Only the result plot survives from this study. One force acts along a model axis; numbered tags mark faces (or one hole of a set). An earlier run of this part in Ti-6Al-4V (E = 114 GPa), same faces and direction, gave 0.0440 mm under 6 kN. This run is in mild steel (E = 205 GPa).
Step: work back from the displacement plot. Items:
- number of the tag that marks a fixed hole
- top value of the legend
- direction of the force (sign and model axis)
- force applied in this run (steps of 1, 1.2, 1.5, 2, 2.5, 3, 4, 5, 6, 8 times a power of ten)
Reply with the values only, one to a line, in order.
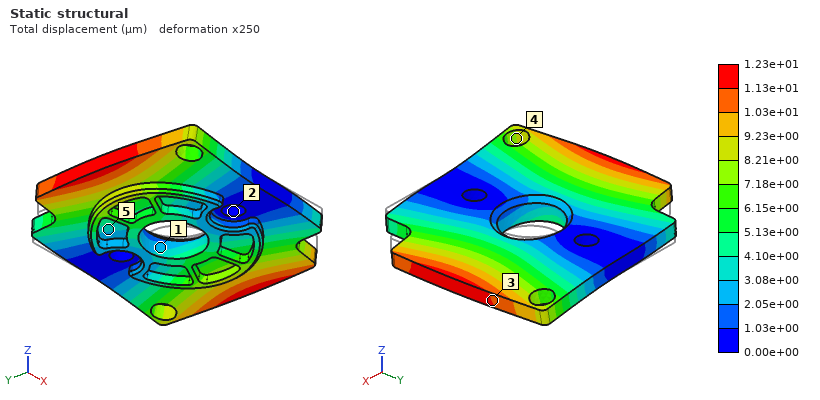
2
1.23e+01 µm
-X
3 kN
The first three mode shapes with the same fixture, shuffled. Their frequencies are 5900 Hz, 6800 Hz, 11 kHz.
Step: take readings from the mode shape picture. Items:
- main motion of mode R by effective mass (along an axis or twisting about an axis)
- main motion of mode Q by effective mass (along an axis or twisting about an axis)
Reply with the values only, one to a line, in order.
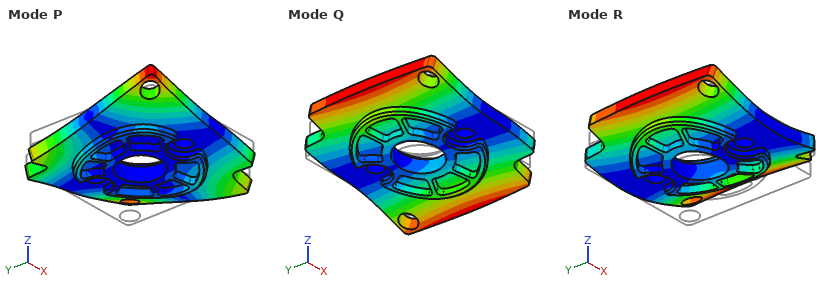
along Z
twisting about Y
